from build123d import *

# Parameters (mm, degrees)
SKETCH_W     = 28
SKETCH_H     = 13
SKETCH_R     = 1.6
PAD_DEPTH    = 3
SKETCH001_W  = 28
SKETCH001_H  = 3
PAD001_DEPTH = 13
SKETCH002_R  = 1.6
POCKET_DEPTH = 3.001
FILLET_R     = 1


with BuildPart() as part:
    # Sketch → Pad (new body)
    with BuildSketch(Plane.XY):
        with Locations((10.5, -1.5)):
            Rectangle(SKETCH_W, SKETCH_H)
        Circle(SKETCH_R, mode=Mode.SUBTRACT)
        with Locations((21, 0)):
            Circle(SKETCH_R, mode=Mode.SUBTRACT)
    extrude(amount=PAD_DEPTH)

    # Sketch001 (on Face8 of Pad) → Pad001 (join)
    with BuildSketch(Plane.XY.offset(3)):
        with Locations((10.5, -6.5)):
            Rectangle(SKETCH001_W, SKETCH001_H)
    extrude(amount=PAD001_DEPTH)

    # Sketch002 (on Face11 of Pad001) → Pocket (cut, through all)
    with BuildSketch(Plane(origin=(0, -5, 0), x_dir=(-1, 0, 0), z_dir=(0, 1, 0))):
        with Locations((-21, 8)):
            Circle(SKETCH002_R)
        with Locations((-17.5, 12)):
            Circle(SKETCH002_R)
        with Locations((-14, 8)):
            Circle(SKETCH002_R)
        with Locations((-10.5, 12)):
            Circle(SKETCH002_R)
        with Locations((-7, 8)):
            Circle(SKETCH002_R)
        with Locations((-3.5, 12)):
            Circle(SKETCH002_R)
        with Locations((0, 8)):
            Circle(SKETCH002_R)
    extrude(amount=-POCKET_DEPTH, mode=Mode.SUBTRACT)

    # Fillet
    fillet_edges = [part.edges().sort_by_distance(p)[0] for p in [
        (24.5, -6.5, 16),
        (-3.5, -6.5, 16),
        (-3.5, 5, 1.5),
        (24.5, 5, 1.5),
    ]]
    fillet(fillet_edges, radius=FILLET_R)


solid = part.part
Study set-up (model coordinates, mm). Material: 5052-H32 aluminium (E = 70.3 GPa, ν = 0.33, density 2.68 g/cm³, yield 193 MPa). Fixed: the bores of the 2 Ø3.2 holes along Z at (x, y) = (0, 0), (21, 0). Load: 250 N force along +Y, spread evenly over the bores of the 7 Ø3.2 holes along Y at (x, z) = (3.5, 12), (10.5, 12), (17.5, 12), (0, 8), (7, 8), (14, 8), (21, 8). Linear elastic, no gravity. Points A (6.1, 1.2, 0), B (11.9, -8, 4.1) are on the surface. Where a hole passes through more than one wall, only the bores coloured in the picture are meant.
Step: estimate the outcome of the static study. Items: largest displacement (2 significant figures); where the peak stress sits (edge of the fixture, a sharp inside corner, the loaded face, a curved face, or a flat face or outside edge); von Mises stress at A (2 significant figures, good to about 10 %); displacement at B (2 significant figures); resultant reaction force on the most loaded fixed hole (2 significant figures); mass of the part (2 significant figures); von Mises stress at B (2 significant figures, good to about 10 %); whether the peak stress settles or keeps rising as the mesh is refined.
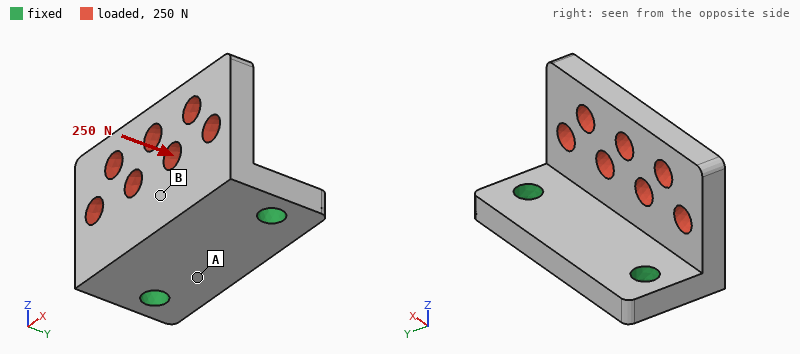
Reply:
68 µm
edge of the fixture
13 MPa
18 µm
130 N
5.3 g
31 MPa
keeps rising
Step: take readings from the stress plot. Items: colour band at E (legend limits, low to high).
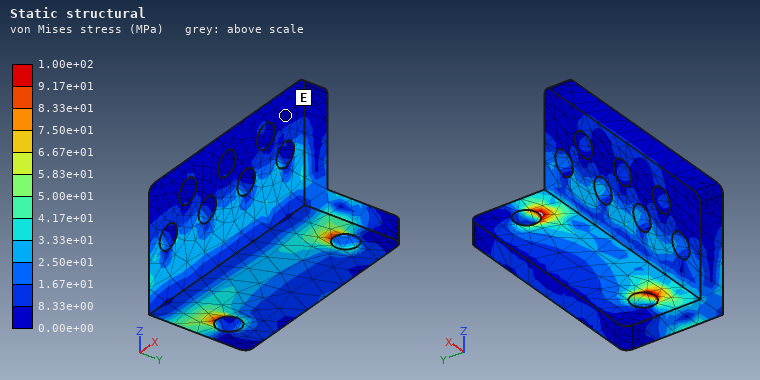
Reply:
0.00e+00 to 8.33e+00 MPa
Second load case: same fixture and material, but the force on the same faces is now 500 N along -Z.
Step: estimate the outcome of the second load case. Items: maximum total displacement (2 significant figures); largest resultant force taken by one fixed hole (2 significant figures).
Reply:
40 µm
250 N
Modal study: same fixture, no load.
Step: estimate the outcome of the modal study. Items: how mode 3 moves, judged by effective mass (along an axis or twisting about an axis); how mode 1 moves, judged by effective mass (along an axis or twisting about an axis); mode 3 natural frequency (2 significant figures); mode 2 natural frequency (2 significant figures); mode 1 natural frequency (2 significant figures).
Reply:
along X
along Y
21 kHz
13 kHz
7300 Hz
